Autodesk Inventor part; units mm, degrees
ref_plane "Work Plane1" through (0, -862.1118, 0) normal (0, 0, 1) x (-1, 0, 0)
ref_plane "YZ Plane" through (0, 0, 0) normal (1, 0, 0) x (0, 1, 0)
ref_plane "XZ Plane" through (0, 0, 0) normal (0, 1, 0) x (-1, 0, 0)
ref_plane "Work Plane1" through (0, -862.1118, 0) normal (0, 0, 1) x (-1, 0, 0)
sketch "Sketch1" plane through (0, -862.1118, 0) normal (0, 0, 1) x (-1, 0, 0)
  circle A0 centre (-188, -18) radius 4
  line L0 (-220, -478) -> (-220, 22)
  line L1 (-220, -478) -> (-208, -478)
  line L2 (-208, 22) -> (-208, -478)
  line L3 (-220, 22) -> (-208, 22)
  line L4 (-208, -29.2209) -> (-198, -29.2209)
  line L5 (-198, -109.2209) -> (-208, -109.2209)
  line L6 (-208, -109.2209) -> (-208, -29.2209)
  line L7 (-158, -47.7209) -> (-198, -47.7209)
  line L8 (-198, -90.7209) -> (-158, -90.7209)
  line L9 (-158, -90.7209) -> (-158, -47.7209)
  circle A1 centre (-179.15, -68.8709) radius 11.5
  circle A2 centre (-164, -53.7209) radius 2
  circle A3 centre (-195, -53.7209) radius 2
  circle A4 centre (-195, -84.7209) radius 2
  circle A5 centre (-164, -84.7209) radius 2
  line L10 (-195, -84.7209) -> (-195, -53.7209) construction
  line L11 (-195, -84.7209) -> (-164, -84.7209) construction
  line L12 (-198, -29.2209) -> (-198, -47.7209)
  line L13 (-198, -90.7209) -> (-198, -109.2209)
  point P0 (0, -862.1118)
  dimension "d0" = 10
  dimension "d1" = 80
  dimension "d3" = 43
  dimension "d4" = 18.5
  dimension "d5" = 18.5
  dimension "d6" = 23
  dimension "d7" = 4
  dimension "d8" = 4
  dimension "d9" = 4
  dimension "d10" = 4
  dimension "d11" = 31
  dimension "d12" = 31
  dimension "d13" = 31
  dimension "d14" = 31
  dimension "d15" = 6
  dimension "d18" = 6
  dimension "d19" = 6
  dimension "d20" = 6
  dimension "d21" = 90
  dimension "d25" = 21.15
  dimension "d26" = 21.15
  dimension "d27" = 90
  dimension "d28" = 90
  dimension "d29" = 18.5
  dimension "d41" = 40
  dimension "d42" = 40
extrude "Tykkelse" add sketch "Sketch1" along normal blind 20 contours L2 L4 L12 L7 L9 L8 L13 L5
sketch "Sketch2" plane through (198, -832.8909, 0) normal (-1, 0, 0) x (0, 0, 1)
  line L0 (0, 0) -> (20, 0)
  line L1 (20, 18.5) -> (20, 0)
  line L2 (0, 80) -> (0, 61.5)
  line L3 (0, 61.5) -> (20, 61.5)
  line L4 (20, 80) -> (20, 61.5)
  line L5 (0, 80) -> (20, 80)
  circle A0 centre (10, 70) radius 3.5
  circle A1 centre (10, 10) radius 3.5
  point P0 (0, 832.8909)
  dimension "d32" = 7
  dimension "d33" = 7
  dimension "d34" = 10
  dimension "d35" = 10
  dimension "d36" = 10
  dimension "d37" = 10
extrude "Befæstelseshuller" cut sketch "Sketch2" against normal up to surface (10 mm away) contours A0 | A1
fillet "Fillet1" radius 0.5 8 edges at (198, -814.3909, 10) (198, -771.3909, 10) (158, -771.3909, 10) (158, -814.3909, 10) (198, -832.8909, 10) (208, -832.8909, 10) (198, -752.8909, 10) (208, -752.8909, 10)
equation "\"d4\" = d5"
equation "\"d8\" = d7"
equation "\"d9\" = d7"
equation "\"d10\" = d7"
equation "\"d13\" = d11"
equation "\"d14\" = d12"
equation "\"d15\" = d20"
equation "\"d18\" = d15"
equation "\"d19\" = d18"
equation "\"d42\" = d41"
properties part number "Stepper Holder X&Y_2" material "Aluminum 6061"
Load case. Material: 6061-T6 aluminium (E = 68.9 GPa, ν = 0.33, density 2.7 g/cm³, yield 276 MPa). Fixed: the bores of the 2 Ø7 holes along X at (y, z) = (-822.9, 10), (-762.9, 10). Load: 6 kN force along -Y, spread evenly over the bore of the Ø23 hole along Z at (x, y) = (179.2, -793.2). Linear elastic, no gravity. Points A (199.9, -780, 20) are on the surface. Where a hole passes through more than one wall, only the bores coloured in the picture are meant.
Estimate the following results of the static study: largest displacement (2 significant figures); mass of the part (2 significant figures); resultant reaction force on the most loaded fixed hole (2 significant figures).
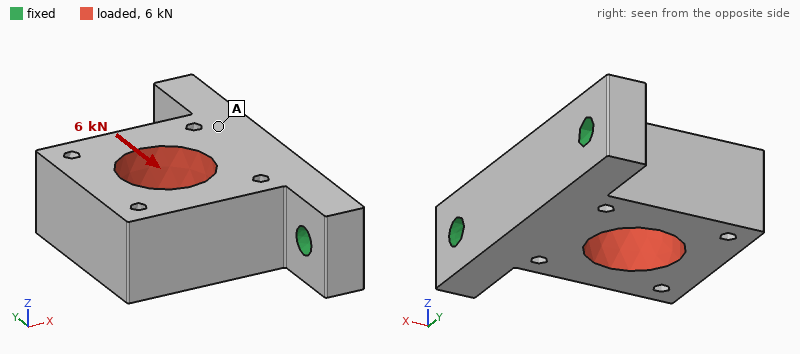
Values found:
49 µm
110 g
4.2 kN
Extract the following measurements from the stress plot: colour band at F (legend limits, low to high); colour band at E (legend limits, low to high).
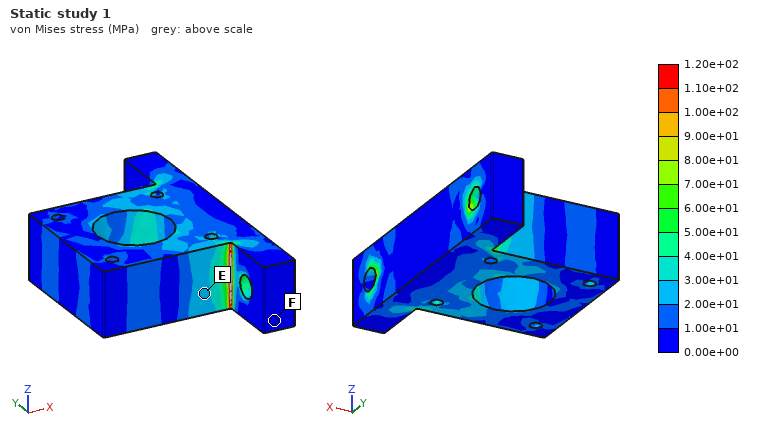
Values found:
0.00e+00 to 1.00e+01 MPa
2.00e+01 to 3.00e+01 MPa
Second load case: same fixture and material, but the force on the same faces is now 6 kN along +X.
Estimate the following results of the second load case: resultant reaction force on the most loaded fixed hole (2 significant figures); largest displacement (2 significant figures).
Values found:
3.2 kN
18 µm
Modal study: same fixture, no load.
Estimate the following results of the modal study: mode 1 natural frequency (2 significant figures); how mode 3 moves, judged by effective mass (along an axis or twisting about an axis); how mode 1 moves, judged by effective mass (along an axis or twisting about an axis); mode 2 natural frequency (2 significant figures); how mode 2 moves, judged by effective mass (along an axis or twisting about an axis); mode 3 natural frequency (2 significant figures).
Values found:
3000 Hz
twisting about X
along Z
7300 Hz
along Y
9500 Hz
